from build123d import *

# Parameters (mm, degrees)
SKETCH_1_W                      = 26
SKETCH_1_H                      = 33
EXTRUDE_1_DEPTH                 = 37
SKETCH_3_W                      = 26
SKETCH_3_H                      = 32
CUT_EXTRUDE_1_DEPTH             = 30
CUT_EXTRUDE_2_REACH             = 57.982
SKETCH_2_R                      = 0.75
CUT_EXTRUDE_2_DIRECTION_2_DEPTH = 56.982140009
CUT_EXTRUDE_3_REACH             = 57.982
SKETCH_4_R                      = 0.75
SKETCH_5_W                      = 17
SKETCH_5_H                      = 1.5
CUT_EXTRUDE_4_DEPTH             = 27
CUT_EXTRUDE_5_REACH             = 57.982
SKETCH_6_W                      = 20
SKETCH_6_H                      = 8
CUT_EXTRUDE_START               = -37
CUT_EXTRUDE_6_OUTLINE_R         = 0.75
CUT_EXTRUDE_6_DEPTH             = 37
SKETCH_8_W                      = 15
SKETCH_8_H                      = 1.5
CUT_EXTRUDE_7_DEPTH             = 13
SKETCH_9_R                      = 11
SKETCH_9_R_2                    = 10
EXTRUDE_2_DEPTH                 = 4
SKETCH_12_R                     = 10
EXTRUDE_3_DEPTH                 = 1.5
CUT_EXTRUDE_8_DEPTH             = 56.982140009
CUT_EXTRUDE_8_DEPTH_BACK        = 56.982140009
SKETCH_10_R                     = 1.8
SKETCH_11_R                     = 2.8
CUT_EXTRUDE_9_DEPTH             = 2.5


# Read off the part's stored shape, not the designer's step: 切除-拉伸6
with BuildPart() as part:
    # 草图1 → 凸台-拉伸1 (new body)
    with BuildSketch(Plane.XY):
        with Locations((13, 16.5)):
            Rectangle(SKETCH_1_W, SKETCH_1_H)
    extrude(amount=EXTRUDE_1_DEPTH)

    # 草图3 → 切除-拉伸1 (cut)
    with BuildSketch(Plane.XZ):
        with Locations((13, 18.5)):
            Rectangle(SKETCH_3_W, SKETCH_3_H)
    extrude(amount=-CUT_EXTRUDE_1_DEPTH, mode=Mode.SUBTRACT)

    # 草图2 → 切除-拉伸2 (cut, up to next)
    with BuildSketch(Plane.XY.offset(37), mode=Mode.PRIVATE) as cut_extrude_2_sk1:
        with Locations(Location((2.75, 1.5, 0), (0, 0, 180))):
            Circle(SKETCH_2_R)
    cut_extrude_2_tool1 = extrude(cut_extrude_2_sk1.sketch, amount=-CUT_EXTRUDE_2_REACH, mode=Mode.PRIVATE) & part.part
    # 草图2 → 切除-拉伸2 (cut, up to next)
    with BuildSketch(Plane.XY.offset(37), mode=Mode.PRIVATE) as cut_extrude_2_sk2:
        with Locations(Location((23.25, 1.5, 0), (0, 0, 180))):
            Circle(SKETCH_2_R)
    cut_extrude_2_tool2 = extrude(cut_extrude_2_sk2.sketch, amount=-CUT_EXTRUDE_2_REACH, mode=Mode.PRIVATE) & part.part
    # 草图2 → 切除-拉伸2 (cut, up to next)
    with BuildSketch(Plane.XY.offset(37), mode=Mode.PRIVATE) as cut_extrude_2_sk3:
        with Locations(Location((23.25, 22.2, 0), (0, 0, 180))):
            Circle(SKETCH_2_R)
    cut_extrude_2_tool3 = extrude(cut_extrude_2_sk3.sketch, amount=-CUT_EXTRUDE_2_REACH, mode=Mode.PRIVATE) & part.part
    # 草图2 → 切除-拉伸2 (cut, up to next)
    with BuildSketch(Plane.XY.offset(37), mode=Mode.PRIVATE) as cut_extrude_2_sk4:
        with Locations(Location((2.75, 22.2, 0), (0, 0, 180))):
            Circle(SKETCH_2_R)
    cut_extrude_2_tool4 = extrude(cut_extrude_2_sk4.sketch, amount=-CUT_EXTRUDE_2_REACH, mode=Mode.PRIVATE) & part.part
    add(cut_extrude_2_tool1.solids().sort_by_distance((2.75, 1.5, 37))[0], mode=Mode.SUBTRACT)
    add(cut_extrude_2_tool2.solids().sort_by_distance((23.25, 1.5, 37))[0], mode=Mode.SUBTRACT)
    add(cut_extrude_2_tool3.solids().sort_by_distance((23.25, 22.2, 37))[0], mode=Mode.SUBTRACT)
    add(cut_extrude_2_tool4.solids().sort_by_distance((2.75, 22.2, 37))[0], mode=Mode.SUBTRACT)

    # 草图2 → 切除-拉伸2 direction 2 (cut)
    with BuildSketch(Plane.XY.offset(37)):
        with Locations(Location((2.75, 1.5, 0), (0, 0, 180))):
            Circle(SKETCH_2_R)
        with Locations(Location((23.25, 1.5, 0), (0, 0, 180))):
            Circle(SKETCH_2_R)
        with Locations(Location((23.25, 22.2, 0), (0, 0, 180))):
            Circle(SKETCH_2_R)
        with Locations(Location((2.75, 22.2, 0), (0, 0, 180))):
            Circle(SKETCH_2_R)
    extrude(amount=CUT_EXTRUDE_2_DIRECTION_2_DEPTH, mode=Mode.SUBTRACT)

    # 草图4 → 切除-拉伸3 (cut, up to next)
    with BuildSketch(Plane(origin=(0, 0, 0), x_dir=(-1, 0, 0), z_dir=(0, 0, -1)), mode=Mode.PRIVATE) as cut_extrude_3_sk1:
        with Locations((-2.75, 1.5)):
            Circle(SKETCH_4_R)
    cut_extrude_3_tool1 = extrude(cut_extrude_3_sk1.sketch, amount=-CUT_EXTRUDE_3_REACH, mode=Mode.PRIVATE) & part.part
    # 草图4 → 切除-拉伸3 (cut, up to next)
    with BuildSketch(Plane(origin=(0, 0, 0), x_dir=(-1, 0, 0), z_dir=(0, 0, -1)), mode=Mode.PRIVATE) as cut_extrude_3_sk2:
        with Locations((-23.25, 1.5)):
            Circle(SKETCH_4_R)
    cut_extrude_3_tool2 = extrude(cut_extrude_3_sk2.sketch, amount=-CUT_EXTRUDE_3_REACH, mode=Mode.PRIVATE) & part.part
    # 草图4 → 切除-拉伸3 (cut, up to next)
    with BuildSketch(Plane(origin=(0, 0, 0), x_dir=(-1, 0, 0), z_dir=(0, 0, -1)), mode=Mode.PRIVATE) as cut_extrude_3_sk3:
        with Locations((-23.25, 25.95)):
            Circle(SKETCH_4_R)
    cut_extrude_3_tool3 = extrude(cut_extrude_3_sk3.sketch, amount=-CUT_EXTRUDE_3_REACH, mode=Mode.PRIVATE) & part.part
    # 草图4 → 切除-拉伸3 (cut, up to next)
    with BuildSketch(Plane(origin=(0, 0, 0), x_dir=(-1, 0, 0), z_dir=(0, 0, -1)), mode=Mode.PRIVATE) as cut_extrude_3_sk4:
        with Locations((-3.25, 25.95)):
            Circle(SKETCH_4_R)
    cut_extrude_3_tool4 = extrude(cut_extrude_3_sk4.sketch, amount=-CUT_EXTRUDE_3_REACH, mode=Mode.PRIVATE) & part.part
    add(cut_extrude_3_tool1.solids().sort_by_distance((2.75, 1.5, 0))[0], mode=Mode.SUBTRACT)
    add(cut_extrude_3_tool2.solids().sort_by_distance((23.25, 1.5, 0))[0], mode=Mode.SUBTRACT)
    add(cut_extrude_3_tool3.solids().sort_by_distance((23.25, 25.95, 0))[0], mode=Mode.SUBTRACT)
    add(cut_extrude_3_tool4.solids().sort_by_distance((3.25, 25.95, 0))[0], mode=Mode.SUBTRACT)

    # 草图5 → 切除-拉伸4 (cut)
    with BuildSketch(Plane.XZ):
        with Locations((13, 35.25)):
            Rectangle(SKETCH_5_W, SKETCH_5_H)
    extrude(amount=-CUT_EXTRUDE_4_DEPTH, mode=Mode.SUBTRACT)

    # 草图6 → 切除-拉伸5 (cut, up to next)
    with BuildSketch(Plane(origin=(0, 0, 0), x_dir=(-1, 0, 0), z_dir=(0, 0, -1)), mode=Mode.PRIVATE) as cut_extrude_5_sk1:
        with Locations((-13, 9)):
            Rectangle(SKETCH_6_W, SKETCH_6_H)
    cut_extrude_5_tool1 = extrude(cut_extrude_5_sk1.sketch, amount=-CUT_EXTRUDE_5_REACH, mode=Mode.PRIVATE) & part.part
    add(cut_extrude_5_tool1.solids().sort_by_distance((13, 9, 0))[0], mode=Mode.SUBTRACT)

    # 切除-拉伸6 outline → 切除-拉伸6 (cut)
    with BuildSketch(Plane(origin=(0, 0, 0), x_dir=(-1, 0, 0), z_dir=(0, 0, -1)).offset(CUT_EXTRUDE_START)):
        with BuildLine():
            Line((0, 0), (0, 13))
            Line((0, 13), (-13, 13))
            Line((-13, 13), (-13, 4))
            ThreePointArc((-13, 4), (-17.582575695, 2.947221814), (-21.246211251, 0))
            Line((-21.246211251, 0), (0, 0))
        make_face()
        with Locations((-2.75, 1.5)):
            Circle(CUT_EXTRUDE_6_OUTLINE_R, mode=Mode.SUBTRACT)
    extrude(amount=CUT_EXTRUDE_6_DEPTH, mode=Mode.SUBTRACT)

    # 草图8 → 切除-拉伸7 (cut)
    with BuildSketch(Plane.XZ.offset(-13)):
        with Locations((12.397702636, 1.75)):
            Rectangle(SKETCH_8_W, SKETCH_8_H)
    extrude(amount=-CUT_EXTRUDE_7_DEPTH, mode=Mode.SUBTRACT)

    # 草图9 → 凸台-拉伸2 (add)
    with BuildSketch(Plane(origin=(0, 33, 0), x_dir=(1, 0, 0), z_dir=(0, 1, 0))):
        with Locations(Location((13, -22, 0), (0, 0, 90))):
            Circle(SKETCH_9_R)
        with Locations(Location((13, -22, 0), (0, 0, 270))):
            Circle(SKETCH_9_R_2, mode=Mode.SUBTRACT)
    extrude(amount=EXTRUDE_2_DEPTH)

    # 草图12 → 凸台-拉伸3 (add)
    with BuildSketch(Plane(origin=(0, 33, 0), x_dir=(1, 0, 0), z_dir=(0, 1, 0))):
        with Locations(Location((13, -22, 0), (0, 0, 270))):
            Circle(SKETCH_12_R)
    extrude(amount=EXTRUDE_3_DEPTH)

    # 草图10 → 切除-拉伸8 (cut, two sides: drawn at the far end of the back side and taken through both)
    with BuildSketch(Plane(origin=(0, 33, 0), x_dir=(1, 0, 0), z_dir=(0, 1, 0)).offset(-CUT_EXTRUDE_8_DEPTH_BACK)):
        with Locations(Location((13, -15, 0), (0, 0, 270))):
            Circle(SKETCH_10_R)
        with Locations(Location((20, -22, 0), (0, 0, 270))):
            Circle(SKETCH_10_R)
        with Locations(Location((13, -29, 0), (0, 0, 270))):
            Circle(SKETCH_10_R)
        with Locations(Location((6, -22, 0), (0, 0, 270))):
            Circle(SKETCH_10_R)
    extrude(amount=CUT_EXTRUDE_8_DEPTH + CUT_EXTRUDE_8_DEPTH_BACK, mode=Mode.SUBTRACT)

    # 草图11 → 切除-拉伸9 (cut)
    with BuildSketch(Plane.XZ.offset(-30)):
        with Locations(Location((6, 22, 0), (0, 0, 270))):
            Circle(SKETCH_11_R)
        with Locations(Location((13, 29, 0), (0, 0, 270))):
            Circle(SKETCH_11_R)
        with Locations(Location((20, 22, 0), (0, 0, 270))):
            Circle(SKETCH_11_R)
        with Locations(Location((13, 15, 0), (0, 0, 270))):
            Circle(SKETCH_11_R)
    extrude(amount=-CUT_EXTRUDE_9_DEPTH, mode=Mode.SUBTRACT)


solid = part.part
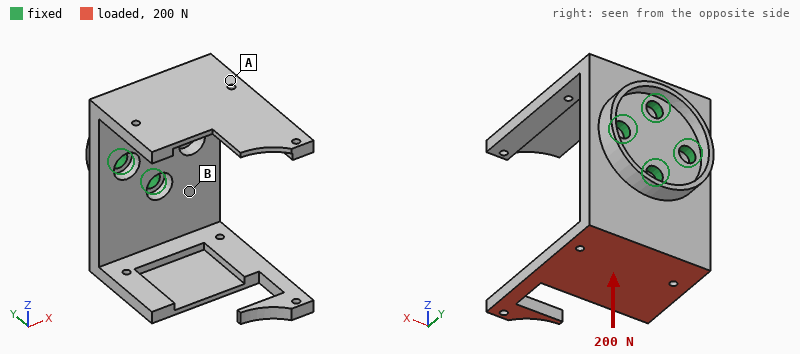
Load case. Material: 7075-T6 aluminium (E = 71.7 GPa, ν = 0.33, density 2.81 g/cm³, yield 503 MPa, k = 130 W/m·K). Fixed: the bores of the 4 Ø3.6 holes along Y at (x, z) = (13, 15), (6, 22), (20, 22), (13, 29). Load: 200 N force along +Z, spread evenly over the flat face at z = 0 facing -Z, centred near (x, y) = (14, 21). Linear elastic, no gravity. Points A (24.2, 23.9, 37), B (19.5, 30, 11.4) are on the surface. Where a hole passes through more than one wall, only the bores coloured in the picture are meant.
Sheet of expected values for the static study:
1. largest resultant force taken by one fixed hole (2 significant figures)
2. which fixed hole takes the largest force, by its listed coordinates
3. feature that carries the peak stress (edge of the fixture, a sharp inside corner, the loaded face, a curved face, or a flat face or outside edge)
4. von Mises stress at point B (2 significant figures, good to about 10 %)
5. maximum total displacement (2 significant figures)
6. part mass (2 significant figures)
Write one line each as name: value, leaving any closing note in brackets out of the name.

largest resultant force taken by one fixed hole: 290 N
which fixed hole takes the largest force, by its listed coordinates: (13, 15)
feature that carries the peak stress: a curved face
von Mises stress at point B: 54 MPa
maximum total displacement: 0.58 mm
part mass: 15 g
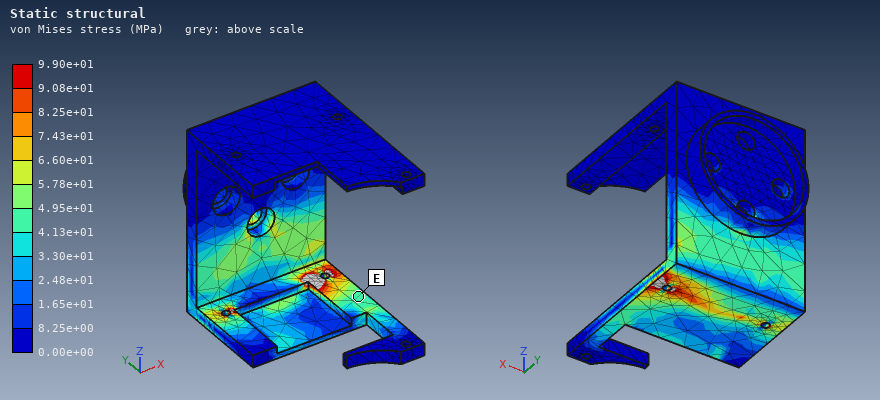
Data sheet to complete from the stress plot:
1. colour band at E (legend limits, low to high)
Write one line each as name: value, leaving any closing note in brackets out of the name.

colour band at E: 4.13e+01 to 4.95e+01 MPa
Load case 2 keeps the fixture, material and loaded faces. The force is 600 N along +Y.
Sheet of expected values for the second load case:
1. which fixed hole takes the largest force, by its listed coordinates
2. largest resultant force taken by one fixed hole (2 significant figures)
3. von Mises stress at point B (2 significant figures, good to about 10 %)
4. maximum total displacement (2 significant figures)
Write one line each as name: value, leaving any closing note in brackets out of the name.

which fixed hole takes the largest force, by its listed coordinates: (13, 15)
largest resultant force taken by one fixed hole: 1.5 kN
von Mises stress at point B: 160 MPa
maximum total displacement: 0.65 mm
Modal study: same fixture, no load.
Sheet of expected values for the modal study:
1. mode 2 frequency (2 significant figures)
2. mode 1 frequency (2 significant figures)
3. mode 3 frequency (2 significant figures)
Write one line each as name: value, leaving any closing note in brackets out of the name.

mode 2 frequency: 2100 Hz
mode 1 frequency: 2100 Hz
mode 3 frequency: 3800 Hz
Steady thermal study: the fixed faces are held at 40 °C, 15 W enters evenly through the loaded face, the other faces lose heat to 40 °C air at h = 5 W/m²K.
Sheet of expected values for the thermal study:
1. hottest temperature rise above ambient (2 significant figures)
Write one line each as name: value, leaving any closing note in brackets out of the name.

hottest temperature rise above ambient: 65 K
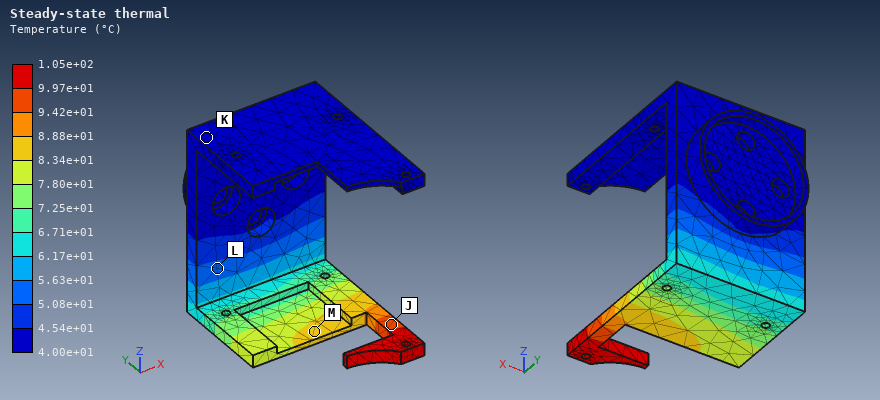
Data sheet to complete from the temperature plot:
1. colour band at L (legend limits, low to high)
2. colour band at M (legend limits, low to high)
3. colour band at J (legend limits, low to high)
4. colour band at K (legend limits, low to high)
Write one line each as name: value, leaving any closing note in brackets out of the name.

colour band at L: 5.08e+01 to 5.63e+01 °C
colour band at M: 8.34e+01 to 8.88e+01 °C
colour band at J: 9.42e+01 to 9.97e+01 °C
colour band at K: 4.00e+01 to 4.54e+01 °C
